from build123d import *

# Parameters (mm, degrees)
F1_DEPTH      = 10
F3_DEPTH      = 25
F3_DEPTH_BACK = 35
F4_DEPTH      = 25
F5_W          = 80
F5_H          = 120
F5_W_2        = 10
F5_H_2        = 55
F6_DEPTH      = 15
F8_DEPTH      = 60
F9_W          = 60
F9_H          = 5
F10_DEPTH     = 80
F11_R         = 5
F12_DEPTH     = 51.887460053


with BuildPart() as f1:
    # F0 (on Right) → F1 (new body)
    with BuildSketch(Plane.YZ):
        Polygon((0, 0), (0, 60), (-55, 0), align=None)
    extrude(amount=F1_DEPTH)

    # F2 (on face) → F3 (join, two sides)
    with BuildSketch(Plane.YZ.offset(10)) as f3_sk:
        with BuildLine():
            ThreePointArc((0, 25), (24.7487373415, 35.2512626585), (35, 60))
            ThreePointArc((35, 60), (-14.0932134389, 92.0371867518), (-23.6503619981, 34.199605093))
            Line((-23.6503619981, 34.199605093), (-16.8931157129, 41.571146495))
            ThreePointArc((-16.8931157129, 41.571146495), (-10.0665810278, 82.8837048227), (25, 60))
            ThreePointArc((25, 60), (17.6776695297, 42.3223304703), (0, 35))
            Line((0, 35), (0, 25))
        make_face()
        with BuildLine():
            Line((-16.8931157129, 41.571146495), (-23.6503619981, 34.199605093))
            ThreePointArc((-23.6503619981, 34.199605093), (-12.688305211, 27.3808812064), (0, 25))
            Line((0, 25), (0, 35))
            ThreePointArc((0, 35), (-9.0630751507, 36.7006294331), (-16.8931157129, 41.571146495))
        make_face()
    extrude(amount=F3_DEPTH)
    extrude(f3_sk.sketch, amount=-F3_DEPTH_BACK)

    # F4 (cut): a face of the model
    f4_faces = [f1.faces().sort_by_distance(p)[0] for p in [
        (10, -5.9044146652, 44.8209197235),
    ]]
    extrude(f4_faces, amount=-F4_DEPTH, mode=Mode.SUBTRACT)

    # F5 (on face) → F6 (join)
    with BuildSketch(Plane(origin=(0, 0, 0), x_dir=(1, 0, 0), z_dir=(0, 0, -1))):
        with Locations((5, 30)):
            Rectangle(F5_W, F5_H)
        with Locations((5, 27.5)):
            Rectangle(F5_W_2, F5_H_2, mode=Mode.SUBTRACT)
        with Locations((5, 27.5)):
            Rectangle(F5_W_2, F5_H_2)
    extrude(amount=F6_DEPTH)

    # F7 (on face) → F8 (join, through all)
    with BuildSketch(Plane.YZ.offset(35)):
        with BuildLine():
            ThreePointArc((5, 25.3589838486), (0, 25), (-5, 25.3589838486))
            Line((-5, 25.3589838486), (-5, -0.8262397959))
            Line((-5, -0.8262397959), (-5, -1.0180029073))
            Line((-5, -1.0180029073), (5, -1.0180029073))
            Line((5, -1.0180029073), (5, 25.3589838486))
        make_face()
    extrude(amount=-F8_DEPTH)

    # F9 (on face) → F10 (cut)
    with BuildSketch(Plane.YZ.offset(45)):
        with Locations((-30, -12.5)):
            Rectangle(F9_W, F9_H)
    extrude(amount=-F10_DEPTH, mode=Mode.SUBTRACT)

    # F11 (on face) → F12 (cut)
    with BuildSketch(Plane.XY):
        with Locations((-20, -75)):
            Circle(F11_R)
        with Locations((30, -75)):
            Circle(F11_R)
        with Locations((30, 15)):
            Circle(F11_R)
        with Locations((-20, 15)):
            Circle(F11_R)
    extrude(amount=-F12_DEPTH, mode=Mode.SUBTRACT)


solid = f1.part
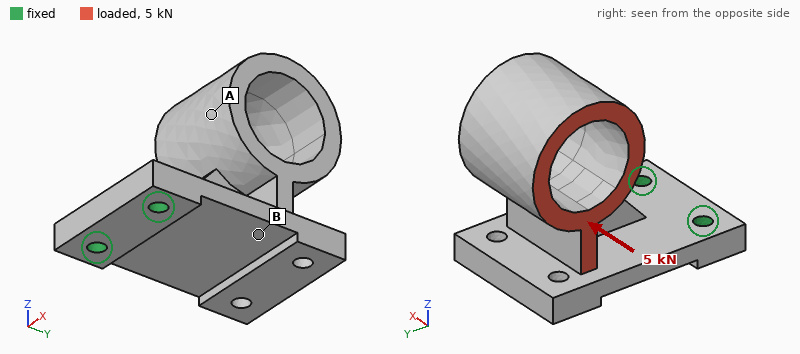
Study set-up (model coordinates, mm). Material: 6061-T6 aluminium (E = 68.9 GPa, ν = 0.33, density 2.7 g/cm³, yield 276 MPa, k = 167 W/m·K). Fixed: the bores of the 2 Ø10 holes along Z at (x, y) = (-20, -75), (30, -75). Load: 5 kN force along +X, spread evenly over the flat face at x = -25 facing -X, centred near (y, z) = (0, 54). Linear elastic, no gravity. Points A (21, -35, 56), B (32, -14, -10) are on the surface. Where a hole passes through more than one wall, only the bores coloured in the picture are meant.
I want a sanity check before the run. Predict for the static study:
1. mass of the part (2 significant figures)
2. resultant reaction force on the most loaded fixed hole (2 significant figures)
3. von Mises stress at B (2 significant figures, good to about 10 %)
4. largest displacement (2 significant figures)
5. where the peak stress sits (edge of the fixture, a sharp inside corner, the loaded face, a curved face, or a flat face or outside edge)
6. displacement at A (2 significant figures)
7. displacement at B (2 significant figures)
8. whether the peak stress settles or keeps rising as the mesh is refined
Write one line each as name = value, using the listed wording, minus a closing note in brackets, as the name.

mass of the part = 690 g
resultant reaction force on the most loaded fixed hole = 9.1 kN
von Mises stress at B = 88 MPa
largest displacement = 1.5 mm
where the peak stress sits = edge of the fixture
displacement at A = 0.84 mm
displacement at B = 0.30 mm
whether the peak stress settles or keeps rising as the mesh is refined = keeps rising
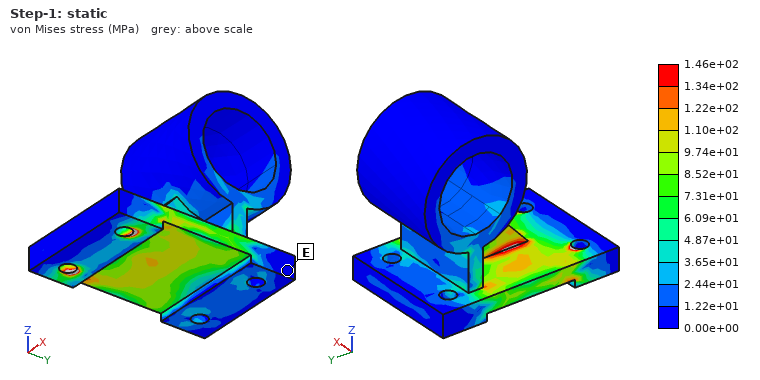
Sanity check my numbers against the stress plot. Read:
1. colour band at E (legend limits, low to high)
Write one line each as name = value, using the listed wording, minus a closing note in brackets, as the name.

colour band at E = 0.00e+00 to 1.22e+01 MPa
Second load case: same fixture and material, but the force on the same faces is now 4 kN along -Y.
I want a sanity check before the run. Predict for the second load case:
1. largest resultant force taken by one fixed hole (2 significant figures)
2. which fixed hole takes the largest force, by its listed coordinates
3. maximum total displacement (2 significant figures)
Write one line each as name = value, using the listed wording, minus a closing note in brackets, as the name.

largest resultant force taken by one fixed hole = 4.3 kN
which fixed hole takes the largest force, by its listed coordinates = (-20, -75)
maximum total displacement = 1.8 mm
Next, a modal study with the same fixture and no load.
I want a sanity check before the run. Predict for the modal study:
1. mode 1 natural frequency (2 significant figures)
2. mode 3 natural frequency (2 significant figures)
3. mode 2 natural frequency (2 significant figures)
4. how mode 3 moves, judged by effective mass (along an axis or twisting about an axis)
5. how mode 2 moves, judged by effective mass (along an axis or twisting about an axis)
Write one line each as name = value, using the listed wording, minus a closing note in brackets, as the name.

mode 1 natural frequency = 360 Hz
mode 3 natural frequency = 1800 Hz
mode 2 natural frequency = 580 Hz
how mode 3 moves, judged by effective mass = along Z
how mode 2 moves, judged by effective mass = along X
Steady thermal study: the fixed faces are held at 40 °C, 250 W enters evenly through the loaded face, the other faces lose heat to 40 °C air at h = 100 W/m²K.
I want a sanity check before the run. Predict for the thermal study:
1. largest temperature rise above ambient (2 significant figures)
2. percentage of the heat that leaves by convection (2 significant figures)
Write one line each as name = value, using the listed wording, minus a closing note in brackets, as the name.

largest temperature rise above ambient = 76 K
percentage of the heat that leaves by convection = 76 %
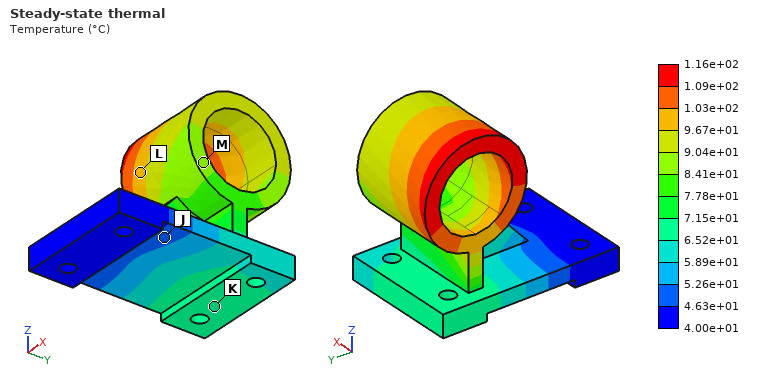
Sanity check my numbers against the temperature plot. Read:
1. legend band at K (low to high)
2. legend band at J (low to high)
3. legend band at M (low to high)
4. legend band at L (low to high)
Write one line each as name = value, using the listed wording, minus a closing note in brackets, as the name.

legend band at K = 6.52e+01 to 7.15e+01 °C
legend band at J = 4.63e+01 to 5.26e+01 °C
legend band at M = 8.41e+01 to 9.04e+01 °C
legend band at L = 9.67e+01 to 1.03e+02 °C
